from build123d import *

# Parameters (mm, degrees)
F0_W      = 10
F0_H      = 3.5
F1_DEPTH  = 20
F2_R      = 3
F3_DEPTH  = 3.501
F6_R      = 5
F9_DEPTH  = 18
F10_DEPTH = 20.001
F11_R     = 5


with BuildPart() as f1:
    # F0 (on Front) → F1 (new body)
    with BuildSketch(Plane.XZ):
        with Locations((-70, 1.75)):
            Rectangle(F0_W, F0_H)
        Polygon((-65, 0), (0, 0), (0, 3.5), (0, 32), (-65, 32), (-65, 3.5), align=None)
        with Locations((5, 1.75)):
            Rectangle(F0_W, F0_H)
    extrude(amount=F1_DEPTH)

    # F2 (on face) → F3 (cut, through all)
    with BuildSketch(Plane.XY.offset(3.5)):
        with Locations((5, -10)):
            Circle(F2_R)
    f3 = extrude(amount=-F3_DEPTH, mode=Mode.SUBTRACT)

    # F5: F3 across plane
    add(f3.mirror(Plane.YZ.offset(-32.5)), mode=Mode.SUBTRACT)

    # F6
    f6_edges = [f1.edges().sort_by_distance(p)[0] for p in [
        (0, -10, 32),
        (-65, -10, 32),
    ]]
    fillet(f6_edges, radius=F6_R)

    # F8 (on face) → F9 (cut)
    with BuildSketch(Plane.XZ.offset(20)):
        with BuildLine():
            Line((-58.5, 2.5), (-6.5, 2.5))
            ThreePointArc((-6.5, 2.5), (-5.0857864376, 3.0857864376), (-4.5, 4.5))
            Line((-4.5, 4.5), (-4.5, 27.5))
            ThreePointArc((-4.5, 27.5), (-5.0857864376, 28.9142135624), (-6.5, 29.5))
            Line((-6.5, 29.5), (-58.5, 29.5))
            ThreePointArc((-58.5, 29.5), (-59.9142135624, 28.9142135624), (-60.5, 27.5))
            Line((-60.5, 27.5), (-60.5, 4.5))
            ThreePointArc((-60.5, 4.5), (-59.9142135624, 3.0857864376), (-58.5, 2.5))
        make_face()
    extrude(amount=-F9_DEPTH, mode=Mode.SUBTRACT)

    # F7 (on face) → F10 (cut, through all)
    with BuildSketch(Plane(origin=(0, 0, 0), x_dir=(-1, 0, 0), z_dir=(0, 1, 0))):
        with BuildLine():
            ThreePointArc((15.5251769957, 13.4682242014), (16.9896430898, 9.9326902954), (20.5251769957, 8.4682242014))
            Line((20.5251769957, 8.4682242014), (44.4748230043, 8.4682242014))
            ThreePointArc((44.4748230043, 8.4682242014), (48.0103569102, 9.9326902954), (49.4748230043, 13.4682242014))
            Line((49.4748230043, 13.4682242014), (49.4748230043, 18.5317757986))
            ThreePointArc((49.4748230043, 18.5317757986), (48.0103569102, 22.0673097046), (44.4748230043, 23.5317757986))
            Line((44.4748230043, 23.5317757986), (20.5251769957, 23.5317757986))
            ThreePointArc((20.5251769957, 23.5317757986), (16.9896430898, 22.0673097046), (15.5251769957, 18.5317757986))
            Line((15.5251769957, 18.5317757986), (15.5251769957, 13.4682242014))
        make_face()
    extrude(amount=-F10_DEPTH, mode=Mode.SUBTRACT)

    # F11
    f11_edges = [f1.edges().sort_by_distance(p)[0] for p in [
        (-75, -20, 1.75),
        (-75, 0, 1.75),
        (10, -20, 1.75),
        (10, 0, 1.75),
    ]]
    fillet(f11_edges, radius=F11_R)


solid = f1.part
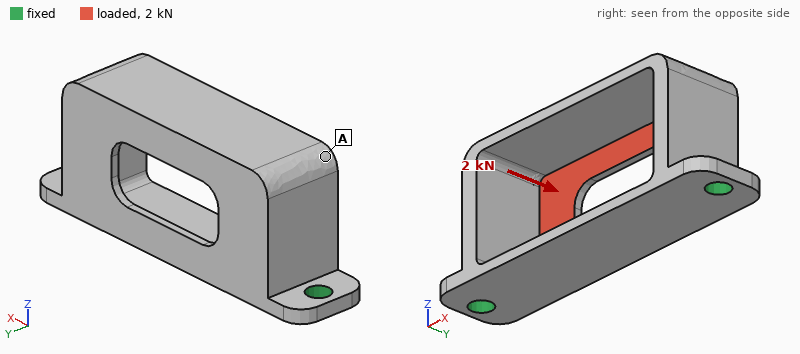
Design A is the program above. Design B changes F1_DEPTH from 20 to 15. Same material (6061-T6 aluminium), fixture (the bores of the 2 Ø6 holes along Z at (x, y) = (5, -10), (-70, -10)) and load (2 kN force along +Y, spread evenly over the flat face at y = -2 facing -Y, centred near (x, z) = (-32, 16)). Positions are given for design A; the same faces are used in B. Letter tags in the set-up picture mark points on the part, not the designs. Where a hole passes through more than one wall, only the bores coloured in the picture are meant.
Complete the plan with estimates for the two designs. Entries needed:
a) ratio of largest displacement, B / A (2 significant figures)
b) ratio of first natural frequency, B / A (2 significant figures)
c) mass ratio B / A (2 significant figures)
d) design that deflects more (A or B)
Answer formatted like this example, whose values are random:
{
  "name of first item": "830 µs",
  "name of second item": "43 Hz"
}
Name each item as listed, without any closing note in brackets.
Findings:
{
  "ratio of largest displacement, B / A": "1.4",
  "ratio of first natural frequency, B / A": "0.96",
  "mass ratio B / A": "0.78",
  "design that deflects more": "B"
}
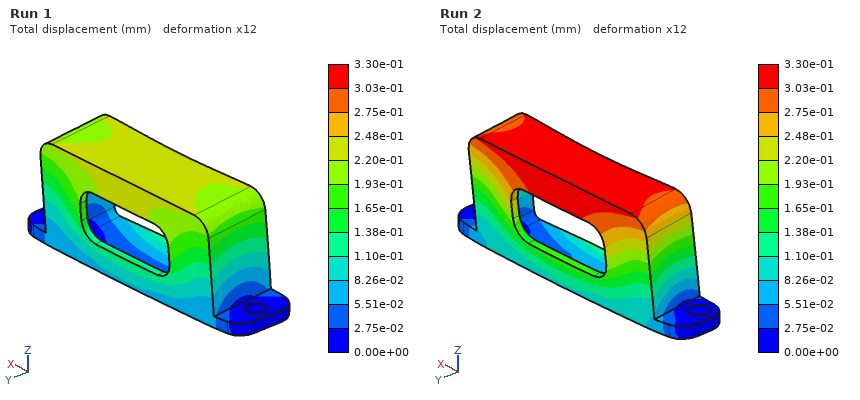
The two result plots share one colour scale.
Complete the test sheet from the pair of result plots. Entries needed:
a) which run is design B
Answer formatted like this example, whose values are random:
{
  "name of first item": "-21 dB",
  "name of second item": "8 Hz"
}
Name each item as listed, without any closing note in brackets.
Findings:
{
  "which run is design B": "Run 2"
}
